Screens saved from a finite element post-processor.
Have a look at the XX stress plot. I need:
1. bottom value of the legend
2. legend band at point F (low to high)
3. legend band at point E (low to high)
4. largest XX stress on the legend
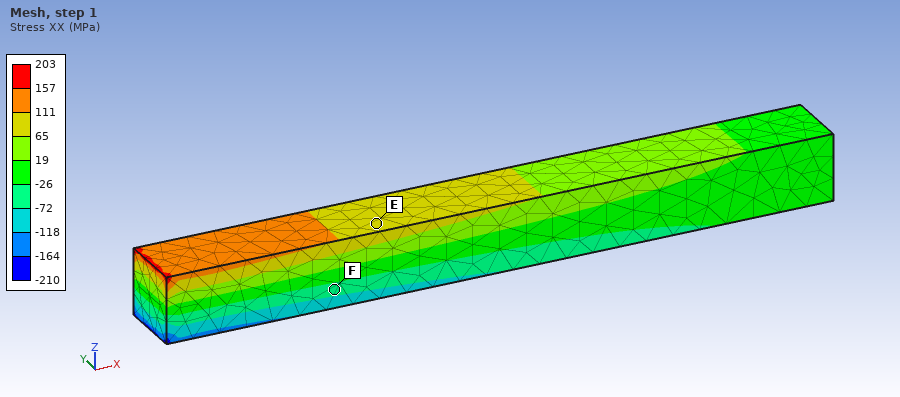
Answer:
-210 MPa
-72 to -26 MPa
65 to 111 MPa
203 MPa
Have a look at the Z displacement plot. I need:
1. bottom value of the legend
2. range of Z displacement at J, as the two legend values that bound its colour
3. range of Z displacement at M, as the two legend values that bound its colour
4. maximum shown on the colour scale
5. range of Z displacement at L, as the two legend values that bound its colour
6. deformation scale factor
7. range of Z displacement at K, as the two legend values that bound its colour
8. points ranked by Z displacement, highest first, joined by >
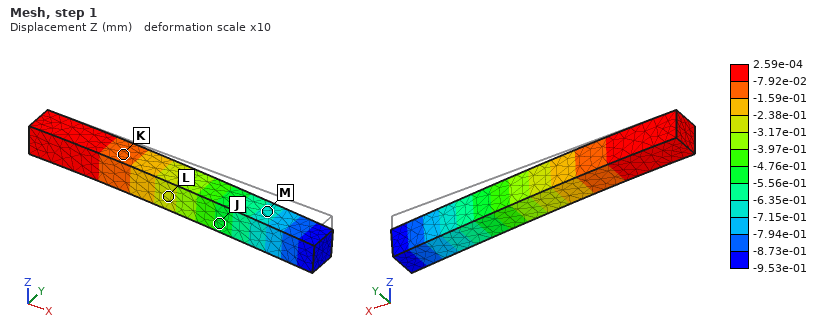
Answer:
-9.53e-01 mm
-5.56e-01 to -4.76e-01 mm
-7.15e-01 to -6.35e-01 mm
2.59e-04 mm
-3.17e-01 to -2.38e-01 mm
10
-1.59e-01 to -7.92e-02 mm
K > L > J > M
